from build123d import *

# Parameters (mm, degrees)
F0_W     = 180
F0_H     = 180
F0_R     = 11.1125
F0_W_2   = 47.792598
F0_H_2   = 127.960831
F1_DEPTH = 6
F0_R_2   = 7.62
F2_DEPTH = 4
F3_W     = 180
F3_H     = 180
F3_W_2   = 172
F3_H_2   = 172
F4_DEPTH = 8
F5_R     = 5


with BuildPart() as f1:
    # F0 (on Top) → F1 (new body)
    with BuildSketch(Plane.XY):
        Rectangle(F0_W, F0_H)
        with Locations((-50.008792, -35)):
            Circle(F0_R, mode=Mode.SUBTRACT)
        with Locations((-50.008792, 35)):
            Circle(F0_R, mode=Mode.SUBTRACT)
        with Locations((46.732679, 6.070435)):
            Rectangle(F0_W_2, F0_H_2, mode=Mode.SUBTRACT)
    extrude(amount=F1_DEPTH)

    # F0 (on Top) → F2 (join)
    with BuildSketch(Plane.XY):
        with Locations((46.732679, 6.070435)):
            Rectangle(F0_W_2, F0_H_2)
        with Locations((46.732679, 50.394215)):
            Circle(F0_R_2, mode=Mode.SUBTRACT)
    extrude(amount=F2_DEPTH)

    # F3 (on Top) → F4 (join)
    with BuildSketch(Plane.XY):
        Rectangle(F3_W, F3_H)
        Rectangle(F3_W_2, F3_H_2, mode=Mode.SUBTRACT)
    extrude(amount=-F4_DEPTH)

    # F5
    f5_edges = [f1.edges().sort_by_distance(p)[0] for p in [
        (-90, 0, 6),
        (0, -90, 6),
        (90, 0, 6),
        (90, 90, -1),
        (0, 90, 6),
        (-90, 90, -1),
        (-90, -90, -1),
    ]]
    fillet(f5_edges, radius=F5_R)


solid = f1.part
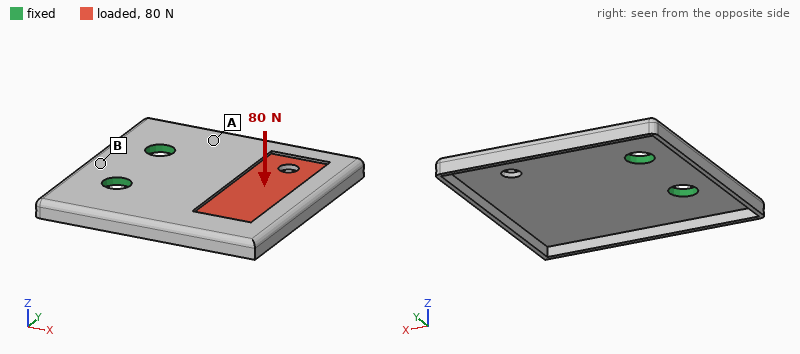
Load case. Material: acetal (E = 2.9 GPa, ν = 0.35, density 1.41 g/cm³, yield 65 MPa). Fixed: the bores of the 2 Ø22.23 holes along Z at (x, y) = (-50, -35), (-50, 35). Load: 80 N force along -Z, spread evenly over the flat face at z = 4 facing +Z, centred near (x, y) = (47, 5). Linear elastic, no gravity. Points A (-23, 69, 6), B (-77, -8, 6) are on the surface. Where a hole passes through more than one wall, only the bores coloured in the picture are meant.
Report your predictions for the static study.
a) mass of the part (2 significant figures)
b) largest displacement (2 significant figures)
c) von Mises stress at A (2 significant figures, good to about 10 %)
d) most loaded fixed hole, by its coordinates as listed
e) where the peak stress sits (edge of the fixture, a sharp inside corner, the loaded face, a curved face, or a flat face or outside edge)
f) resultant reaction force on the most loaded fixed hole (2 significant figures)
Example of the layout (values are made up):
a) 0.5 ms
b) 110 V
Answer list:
a) 280 g
b) 2.7 mm
c) 3.0 MPa
d) (-50, 35)
e) a flat face or outside edge
f) 44 N
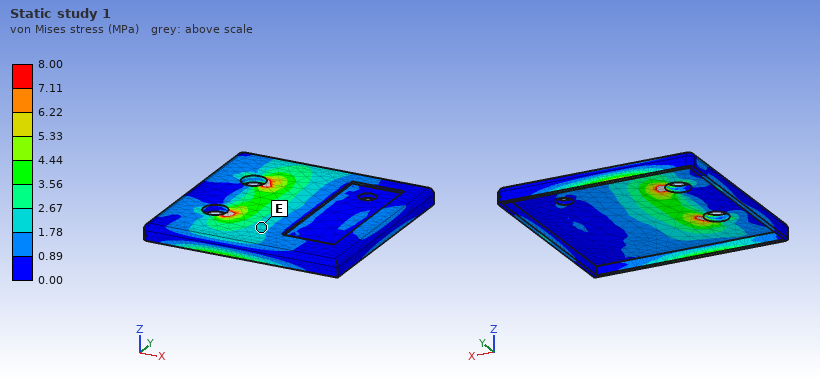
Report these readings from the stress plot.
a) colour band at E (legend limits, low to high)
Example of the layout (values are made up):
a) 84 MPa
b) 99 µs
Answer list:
a) 1.78 to 2.67 MPa
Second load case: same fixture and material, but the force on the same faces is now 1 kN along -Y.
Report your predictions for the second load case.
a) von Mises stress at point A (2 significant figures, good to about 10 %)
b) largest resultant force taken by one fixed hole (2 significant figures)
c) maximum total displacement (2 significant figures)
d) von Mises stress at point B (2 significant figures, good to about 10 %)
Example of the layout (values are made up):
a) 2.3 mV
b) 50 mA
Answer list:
a) 1.2 MPa
b) 1.2 kN
c) 0.62 mm
d) 0.93 MPa
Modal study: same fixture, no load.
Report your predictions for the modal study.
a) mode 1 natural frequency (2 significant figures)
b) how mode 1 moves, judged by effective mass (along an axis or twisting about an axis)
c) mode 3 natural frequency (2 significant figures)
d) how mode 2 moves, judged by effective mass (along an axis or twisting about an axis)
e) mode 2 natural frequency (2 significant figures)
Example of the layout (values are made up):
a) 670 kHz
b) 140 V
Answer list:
a) 88 Hz
b) along Z
c) 370 Hz
d) twisting about X
e) 130 Hz
